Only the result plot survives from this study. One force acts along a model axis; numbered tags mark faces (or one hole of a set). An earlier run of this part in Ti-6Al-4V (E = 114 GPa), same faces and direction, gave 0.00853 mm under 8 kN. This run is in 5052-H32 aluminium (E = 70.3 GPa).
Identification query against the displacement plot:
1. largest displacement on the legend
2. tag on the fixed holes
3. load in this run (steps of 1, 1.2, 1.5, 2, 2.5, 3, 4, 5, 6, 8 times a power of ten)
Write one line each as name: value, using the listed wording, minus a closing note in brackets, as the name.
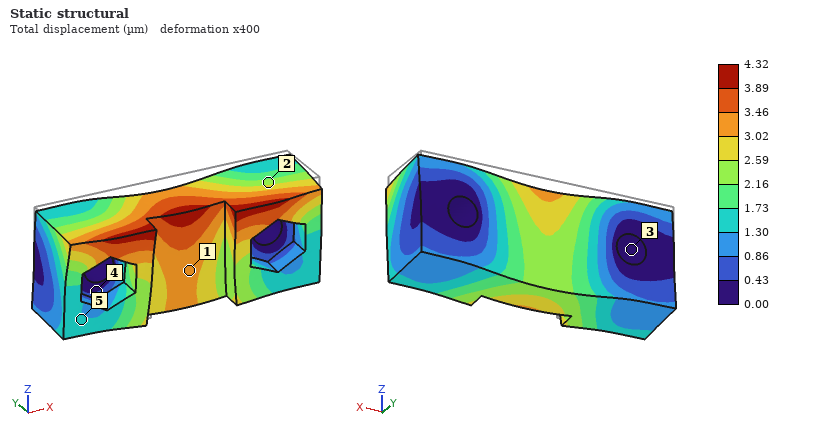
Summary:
largest displacement on the legend: 4.32 µm
tag on the fixed holes: 3
load in this run: 2.5 kN
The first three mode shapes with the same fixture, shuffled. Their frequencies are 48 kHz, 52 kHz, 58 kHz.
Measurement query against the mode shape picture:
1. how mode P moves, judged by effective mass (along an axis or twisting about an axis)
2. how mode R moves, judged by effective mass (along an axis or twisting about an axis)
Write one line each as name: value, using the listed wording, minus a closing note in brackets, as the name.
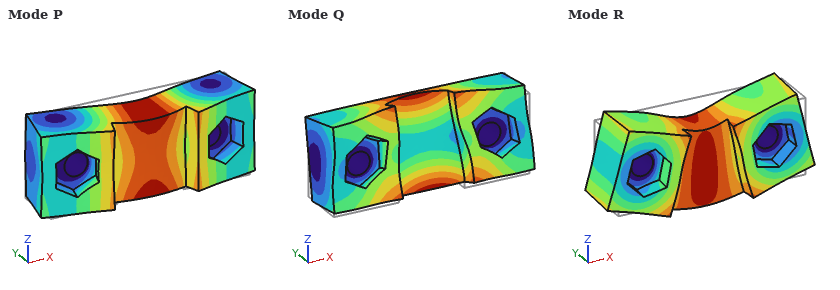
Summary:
how mode P moves, judged by effective mass: along Y
how mode R moves, judged by effective mass: along Z
